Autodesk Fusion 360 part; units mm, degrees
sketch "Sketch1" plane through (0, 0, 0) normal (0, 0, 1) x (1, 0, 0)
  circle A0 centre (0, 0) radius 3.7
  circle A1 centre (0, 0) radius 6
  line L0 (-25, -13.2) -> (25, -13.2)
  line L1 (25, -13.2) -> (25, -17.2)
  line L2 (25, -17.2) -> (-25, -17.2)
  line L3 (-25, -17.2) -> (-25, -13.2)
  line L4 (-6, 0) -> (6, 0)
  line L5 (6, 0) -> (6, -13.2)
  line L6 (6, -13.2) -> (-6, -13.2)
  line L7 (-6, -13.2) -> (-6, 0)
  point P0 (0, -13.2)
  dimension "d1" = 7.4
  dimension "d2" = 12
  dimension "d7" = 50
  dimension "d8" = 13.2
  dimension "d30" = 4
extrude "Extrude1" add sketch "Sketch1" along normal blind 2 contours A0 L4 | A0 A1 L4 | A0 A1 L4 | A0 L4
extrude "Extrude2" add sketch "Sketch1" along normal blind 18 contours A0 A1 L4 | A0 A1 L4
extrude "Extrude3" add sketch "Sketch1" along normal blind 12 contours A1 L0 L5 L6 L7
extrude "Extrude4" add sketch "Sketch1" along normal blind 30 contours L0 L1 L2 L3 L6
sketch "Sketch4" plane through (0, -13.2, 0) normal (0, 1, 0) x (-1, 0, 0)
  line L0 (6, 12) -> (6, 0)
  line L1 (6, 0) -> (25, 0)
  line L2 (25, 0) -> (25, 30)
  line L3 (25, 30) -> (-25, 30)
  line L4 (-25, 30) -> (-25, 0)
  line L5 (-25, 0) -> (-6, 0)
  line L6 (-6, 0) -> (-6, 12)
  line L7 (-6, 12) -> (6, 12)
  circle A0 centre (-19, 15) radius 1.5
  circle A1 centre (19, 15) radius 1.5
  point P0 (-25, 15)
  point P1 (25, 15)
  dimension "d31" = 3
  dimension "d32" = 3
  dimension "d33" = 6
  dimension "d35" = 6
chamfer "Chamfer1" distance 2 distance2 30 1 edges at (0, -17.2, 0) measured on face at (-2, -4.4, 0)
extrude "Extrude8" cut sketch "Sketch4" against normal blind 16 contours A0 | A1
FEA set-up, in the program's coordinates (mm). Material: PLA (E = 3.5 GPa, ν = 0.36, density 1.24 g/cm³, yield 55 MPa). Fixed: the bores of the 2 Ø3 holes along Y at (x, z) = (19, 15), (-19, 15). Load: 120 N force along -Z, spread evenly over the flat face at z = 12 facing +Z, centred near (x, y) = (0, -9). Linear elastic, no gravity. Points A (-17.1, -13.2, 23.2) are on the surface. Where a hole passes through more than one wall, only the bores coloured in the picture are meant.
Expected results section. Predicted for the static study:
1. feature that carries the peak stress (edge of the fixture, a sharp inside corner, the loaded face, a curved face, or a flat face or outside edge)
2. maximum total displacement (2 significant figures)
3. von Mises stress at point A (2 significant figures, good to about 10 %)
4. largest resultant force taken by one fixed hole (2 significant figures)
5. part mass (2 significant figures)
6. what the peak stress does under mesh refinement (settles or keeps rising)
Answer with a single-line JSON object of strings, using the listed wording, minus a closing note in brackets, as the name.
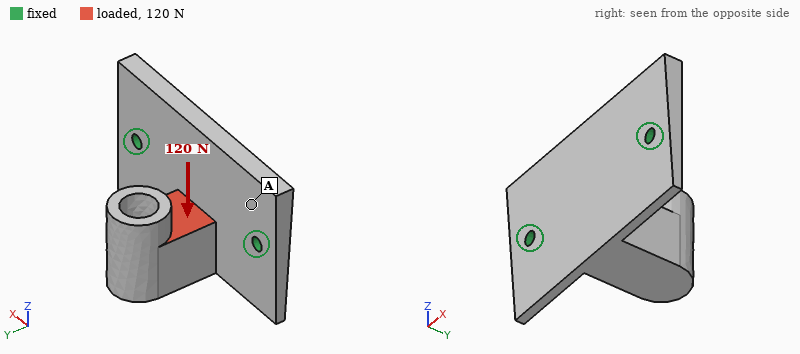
{"feature that carries the peak stress": "edge of the fixture", "maximum total displacement": "0.65 mm", "von Mises stress at point A": "2.9 MPa", "largest resultant force taken by one fixed hole": "60 N", "part mass": "8.7 g", "what the peak stress does under mesh refinement": "keeps rising"}
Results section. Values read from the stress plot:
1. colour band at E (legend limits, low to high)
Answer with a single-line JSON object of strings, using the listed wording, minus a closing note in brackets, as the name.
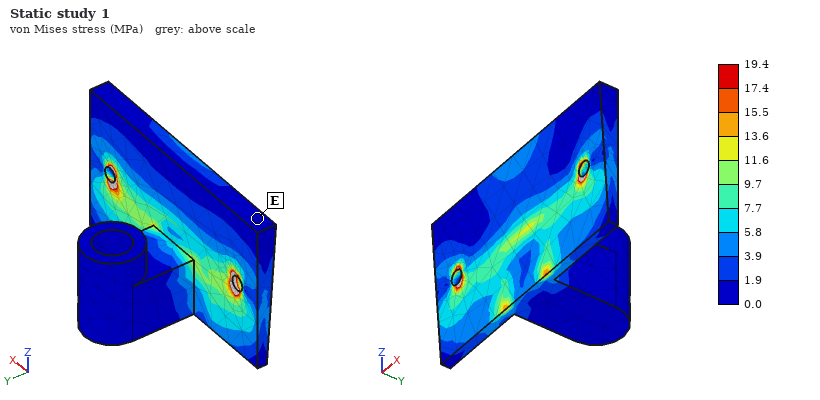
{"colour band at E": "0.0 to 1.9 MPa"}
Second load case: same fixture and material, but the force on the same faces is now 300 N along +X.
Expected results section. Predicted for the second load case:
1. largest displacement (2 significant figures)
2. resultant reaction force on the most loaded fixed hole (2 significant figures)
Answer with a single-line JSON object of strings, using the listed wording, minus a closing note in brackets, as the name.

{"largest displacement": "0.44 mm", "resultant reaction force on the most loaded fixed hole": "160 N"}
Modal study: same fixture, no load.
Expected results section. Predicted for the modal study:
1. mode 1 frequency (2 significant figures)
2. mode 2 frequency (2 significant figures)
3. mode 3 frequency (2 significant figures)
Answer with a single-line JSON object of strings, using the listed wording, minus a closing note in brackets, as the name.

{"mode 1 frequency": "950 Hz", "mode 2 frequency": "2100 Hz", "mode 3 frequency": "2100 Hz"}
